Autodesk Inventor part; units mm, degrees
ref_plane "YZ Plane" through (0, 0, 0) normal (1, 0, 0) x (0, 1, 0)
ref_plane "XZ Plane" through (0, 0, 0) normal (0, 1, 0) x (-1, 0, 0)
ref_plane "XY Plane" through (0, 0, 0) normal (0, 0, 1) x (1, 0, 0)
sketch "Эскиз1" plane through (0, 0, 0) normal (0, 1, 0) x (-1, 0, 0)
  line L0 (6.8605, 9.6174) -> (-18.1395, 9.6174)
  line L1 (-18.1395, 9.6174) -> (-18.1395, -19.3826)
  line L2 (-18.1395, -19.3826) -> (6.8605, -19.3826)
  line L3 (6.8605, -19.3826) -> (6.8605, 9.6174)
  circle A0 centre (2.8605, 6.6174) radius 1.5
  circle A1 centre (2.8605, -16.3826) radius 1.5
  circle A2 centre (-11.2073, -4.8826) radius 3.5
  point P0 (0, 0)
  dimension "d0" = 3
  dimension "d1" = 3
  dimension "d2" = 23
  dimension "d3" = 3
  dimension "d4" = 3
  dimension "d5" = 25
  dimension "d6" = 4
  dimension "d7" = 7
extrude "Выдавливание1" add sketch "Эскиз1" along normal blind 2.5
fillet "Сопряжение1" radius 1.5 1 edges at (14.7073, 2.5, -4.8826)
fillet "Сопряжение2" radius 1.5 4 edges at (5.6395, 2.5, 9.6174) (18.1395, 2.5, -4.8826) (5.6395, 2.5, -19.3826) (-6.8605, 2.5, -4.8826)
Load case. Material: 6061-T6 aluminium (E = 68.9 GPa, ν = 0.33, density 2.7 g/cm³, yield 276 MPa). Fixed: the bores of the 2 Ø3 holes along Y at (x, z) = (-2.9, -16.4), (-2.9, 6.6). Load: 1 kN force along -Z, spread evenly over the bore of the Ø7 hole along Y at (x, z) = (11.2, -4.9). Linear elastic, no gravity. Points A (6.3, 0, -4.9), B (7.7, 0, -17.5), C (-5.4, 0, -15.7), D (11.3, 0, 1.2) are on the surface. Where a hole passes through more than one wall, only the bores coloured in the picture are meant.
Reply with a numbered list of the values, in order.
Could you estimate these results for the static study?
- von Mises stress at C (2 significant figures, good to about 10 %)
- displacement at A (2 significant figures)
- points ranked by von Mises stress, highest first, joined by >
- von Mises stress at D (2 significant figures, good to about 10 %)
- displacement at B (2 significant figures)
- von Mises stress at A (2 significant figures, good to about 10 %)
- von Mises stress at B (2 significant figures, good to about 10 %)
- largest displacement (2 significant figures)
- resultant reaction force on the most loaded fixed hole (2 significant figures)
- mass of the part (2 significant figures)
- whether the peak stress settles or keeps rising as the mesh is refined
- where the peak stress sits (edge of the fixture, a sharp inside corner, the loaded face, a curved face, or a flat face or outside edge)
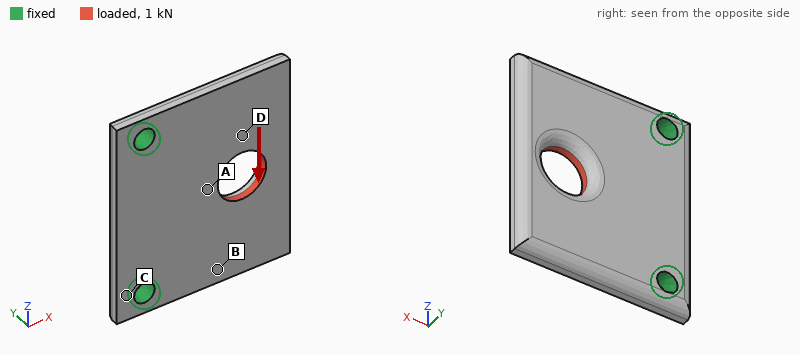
1. 10 MPa
2. 8.8 µm
3. A > D > B > C
4. 53 MPa
5. 14 µm
6. 68 MPa
7. 21 MPa
8. 34 µm
9. 760 N
10. 4.4 g
11. keeps rising
12. edge of the fixture
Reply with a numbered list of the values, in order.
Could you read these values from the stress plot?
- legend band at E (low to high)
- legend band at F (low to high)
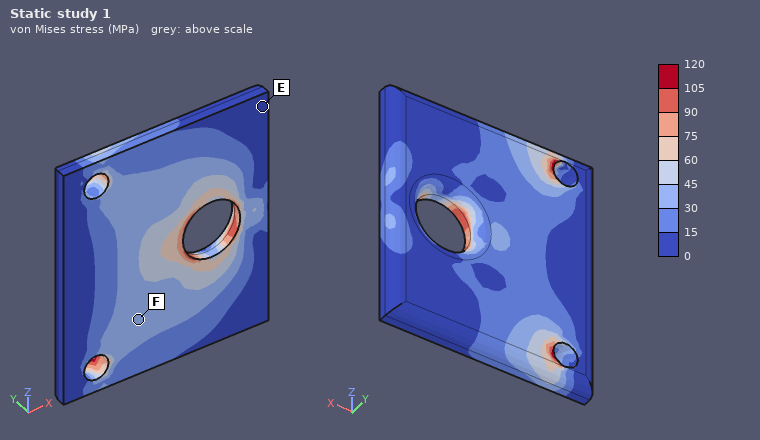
1. 0 to 15 MPa
2. 30 to 45 MPa
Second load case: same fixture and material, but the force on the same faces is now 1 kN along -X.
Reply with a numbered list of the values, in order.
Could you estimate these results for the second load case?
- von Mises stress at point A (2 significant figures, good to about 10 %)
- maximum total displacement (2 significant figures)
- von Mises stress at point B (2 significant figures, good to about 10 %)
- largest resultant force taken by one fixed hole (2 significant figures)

1. 47 MPa
2. 73 µm
3. 28 MPa
4. 530 N
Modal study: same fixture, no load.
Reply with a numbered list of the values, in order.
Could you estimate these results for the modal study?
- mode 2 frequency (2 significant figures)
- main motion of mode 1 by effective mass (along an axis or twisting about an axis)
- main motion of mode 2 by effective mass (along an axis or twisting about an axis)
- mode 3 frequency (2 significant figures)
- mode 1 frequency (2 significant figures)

1. 8700 Hz
2. along Y
3. twisting about X
4. 18 kHz
5. 4500 Hz
